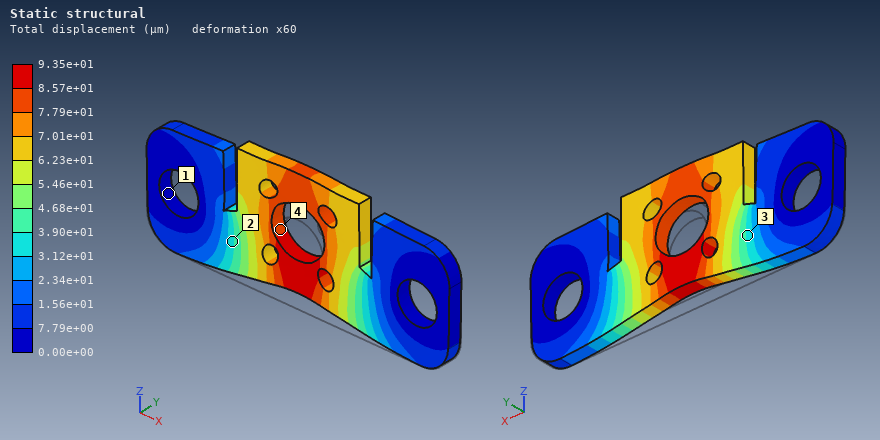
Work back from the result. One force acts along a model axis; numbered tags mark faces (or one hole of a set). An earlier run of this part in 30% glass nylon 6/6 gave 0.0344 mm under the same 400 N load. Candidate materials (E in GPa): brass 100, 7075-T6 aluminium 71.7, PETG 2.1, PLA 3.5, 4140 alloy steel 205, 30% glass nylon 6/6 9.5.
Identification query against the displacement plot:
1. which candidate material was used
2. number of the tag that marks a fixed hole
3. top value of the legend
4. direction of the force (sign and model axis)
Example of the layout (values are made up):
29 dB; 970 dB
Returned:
PLA; 1; 9.35e+01 µm; +Z
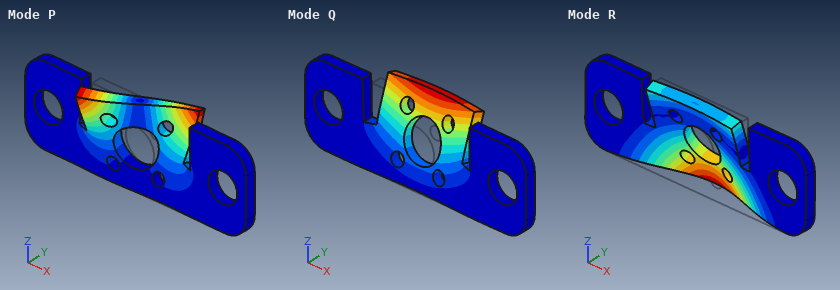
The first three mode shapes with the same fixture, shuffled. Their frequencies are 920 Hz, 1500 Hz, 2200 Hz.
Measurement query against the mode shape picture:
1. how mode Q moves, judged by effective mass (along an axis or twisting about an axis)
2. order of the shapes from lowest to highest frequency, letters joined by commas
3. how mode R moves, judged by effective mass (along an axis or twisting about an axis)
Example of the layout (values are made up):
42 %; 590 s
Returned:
along Y; Q, R, P; along Y
